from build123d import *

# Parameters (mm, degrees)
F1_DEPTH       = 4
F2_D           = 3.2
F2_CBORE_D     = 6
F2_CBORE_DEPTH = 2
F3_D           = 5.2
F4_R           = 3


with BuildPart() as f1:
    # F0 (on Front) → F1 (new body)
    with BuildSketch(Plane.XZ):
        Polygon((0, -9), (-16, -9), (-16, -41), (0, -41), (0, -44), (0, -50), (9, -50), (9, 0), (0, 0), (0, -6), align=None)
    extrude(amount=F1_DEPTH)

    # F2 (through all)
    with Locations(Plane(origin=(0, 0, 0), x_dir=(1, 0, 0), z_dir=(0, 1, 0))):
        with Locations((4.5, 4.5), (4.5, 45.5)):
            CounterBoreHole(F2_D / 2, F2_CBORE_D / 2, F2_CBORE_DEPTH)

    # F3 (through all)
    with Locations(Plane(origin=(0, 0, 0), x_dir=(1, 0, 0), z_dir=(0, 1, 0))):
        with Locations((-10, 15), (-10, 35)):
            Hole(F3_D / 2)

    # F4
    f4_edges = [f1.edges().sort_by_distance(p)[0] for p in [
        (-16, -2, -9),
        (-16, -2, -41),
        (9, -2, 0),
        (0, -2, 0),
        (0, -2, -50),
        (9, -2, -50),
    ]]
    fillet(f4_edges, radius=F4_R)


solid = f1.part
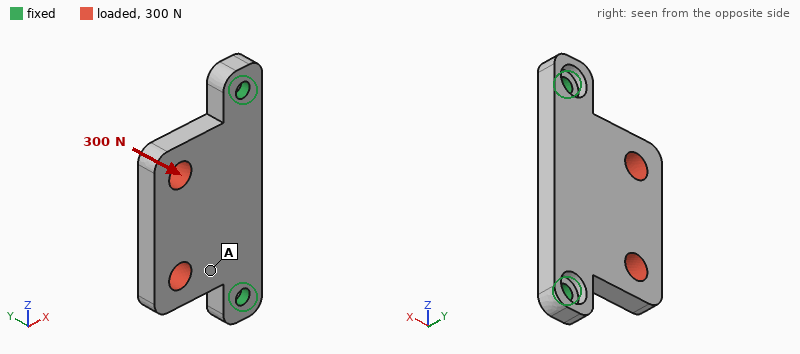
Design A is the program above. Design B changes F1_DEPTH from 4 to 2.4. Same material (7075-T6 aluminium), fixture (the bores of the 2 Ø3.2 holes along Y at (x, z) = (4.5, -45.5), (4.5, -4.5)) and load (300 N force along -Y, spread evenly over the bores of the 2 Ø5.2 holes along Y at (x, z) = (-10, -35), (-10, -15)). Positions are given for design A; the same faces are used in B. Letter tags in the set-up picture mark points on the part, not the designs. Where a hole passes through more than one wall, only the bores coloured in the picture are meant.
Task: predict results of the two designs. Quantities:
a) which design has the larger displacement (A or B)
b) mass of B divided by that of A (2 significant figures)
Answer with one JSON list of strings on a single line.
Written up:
["B", "0.59"]
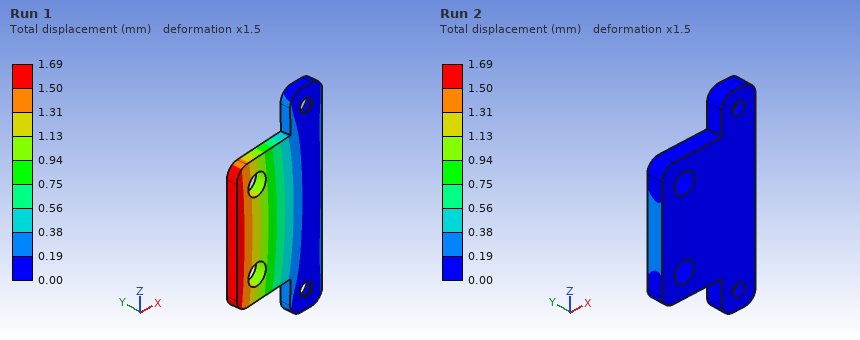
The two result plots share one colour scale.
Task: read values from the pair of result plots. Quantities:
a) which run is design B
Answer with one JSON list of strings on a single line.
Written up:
["Run 1"]
